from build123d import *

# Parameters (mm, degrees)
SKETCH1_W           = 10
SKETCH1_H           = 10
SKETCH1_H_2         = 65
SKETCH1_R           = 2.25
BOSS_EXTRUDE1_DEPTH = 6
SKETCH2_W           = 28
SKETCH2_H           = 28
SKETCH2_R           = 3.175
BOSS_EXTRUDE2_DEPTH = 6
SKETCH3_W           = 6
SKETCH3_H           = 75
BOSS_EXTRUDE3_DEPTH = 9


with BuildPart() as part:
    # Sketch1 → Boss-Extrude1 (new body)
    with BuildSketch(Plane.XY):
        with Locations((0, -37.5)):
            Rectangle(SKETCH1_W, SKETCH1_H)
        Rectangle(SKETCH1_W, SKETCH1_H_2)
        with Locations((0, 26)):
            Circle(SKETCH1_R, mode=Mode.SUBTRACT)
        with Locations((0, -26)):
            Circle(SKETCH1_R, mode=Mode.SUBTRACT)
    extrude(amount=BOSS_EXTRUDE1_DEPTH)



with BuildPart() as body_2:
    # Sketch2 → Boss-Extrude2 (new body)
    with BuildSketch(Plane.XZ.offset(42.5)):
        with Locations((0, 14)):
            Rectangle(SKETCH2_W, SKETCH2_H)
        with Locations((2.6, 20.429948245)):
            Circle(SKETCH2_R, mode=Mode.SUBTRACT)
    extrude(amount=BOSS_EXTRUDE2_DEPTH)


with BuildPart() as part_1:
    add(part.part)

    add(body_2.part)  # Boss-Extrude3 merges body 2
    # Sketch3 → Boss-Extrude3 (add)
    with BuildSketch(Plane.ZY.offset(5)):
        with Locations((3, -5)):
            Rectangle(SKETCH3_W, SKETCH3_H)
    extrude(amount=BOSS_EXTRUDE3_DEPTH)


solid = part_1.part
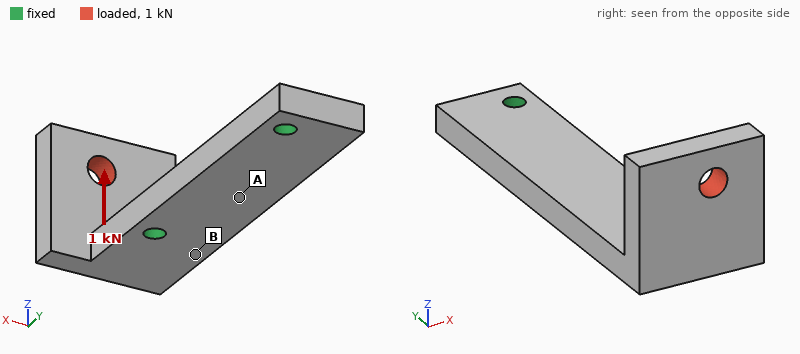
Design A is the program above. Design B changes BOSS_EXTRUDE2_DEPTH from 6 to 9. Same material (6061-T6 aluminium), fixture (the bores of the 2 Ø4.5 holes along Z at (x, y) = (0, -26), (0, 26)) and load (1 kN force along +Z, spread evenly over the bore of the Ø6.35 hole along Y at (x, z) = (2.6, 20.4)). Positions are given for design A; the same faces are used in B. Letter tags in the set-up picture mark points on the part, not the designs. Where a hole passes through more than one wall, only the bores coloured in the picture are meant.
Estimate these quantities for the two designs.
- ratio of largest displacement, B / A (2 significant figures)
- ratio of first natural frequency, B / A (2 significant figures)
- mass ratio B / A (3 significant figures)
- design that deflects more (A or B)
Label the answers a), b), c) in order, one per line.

a) 1.2
b) 0.79
c) 1.18
d) B
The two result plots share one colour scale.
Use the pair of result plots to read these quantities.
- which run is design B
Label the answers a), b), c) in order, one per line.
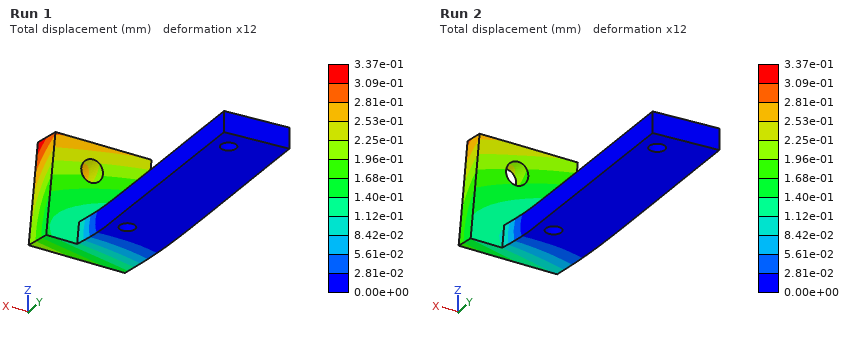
a) Run 1
